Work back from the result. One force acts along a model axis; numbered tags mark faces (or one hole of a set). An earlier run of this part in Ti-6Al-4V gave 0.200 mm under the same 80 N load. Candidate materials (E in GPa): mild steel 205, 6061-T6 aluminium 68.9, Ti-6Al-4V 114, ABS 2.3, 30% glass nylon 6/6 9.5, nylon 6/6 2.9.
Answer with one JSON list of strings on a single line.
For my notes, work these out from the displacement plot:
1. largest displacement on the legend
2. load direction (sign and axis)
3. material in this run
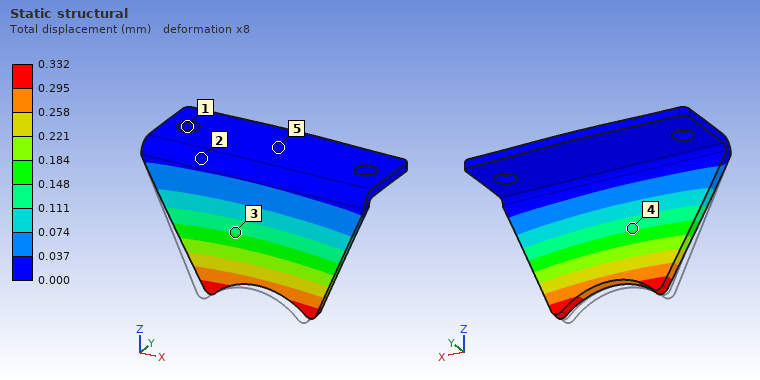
["0.332 mm", "+Y", "6061-T6 aluminium"]
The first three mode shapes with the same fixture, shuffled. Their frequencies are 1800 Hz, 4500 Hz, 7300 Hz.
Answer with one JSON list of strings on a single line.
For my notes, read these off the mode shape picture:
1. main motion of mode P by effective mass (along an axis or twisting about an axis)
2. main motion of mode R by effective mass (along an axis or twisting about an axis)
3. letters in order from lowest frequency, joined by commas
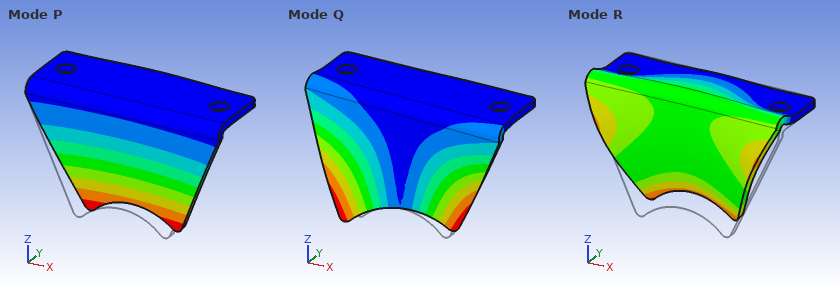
["along Y", "along Z", "P, Q, R"]
